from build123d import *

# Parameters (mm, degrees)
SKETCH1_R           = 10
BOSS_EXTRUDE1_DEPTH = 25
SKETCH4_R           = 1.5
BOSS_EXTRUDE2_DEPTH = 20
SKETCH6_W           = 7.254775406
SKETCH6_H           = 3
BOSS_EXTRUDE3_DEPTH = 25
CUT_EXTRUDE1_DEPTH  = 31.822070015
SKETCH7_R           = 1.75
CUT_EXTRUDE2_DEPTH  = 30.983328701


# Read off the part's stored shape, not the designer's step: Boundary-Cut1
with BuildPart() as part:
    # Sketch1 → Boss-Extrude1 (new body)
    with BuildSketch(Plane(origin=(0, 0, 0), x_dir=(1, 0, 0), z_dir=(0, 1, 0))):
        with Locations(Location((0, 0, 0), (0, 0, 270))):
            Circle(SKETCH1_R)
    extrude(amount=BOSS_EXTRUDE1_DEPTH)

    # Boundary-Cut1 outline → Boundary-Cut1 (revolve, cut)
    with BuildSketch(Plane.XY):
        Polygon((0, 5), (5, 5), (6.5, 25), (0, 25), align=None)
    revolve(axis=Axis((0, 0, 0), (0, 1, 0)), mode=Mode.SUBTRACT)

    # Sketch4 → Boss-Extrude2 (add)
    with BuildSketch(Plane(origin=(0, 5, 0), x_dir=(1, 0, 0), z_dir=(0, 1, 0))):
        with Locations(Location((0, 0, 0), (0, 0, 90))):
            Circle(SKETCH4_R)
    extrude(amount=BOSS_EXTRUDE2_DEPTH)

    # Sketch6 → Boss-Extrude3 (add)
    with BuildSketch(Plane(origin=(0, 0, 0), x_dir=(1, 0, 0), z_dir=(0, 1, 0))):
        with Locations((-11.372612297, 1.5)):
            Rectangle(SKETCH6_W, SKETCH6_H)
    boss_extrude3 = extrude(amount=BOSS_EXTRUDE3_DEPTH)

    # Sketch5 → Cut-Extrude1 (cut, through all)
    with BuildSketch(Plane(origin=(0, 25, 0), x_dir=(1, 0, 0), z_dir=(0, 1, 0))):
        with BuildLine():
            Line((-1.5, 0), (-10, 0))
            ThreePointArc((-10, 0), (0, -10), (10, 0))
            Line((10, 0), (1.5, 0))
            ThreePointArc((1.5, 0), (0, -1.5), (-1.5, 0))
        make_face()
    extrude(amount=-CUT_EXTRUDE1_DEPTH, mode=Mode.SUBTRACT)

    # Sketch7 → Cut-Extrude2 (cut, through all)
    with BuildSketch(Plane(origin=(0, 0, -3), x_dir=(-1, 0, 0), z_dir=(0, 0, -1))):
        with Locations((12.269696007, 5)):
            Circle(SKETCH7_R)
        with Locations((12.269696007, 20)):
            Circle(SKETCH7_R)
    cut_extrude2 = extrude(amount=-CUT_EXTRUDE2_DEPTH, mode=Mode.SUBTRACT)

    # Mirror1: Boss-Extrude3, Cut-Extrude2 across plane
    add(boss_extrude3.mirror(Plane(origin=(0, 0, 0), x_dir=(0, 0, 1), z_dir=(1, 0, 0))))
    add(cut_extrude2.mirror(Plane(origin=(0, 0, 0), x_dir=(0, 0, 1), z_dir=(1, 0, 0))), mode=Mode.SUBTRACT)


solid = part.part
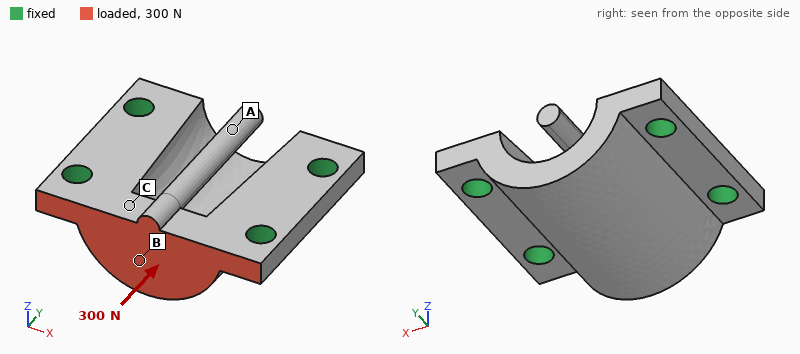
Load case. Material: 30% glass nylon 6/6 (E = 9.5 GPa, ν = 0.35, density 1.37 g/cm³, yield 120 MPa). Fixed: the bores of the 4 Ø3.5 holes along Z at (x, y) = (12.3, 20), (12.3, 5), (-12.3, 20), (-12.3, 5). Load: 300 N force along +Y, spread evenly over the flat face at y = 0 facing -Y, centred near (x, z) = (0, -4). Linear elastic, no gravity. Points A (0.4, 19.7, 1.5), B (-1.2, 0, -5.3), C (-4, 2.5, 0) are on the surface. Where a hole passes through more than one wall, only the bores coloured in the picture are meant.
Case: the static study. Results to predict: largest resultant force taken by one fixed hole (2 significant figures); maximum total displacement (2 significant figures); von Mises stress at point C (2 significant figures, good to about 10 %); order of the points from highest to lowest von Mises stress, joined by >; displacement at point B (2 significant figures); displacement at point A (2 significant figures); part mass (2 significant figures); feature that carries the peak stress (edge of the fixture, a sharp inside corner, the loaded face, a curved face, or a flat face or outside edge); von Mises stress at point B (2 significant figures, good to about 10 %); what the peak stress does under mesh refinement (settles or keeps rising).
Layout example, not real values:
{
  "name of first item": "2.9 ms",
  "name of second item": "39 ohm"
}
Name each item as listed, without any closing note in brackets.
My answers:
{
  "largest resultant force taken by one fixed hole": "100 N",
  "maximum total displacement": "11 µm",
  "von Mises stress at point C": "3.6 MPa",
  "order of the points from highest to lowest von Mises stress, joined by >": "C > B > A",
  "displacement at point B": "6.7 µm",
  "displacement at point A": "10 µm",
  "part mass": "5.1 g",
  "feature that carries the peak stress": "edge of the fixture",
  "von Mises stress at point B": "2.4 MPa",
  "what the peak stress does under mesh refinement": "keeps rising"
}
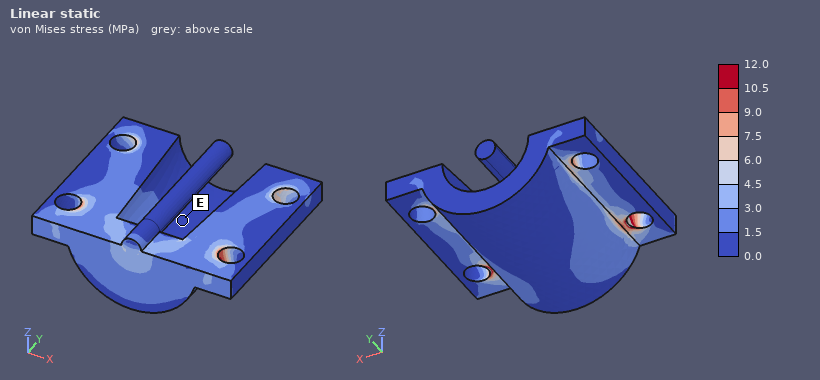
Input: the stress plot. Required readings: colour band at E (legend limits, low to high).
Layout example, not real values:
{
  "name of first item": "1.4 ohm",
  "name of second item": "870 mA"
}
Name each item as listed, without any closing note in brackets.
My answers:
{
  "colour band at E": "0.0 to 1.5 MPa"
}
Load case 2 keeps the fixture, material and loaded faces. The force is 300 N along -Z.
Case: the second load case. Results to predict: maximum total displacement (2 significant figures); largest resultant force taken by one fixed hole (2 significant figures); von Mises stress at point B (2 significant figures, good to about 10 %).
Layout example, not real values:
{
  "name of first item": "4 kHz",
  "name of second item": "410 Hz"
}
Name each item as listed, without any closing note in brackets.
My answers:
{
  "maximum total displacement": "45 µm",
  "largest resultant force taken by one fixed hole": "210 N",
  "von Mises stress at point B": "6.1 MPa"
}
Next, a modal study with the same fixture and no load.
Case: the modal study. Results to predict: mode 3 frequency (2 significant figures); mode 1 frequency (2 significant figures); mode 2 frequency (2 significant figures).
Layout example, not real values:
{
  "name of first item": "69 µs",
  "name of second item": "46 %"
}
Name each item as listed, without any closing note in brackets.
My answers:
{
  "mode 3 frequency": "14 kHz",
  "mode 1 frequency": "2400 Hz",
  "mode 2 frequency": "2400 Hz"
}
